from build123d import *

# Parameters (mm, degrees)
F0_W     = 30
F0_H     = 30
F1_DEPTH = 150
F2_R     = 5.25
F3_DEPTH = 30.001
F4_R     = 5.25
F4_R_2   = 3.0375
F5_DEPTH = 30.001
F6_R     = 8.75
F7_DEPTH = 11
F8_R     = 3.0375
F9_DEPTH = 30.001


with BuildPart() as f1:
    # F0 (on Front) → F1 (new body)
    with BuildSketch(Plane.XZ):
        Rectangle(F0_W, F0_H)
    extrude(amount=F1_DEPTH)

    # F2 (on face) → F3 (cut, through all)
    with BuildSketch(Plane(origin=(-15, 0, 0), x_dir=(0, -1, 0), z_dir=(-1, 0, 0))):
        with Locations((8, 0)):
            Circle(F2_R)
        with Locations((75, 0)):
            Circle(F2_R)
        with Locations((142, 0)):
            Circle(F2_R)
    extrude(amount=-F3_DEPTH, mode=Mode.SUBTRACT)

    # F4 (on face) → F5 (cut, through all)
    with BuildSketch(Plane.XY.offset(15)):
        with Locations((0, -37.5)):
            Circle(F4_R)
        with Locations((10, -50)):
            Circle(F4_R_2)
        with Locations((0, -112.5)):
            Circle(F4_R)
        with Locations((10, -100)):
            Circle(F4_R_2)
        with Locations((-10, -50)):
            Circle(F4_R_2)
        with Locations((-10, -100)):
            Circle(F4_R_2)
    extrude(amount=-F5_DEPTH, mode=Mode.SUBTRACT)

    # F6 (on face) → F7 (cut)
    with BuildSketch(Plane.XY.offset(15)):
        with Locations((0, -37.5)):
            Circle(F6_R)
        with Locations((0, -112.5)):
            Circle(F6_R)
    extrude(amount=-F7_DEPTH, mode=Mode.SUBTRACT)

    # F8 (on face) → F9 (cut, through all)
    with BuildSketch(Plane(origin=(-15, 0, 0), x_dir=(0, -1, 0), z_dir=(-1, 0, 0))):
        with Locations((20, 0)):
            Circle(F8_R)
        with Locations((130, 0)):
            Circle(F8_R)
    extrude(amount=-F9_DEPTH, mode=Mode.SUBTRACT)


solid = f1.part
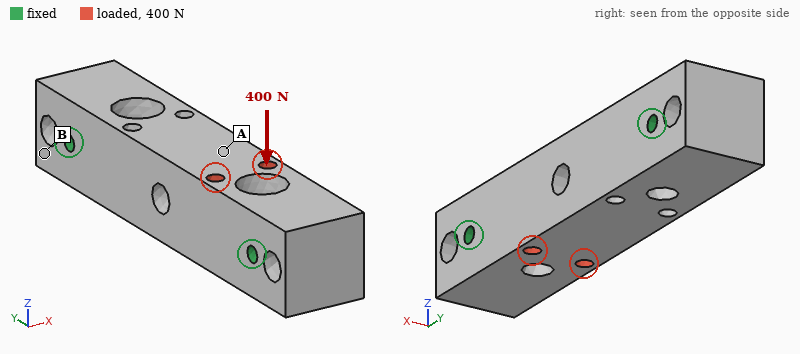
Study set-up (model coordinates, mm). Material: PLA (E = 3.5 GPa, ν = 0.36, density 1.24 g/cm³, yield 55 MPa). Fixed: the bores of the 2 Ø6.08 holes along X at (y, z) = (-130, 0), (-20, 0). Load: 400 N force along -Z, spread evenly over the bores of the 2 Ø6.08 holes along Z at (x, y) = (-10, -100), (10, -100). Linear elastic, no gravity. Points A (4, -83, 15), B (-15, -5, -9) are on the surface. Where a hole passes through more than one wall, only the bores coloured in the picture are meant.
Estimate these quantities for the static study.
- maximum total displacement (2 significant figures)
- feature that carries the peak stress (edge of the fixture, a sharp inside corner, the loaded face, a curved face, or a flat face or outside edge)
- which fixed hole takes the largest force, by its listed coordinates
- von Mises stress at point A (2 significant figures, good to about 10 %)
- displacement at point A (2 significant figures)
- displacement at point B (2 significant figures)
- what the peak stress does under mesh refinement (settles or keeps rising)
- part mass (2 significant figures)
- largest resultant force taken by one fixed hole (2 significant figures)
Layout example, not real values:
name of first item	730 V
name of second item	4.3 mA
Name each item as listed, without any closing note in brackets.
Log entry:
maximum total displacement	35 µm
feature that carries the peak stress	a sharp inside corner
which fixed hole takes the largest force, by its listed coordinates	(-130, 0)
von Mises stress at point A	0.97 MPa
displacement at point A	32 µm
displacement at point B	6.6 µm
what the peak stress does under mesh refinement	keeps rising
part mass	140 g
largest resultant force taken by one fixed hole	310 N
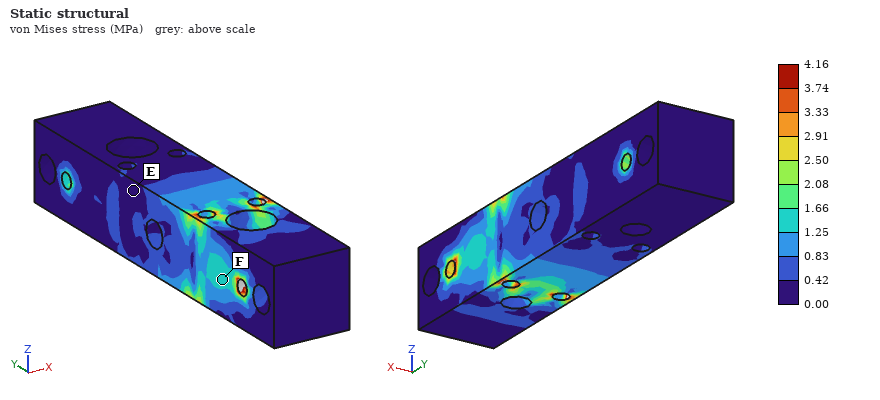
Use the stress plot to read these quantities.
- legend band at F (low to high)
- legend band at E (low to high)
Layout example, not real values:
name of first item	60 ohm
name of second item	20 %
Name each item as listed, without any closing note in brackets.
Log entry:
legend band at F	1.25 to 1.66 MPa
legend band at E	0.00 to 0.42 MPa
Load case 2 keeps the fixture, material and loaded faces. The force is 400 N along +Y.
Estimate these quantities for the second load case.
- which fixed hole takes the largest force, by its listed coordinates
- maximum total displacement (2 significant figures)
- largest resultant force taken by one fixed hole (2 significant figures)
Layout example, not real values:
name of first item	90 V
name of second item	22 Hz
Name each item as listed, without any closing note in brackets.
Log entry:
which fixed hole takes the largest force, by its listed coordinates	(-130, 0)
maximum total displacement	5.3 µm
largest resultant force taken by one fixed hole	280 N
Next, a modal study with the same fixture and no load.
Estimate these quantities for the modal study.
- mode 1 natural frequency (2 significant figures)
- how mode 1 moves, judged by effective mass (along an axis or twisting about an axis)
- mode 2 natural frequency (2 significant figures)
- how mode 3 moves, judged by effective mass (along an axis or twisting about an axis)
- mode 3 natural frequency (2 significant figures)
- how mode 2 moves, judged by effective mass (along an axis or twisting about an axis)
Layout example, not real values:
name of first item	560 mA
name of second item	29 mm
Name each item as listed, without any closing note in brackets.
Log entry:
mode 1 natural frequency	2100 Hz
how mode 1 moves, judged by effective mass	along Z
mode 2 natural frequency	2400 Hz
how mode 3 moves, judged by effective mass	twisting about Y
mode 3 natural frequency	3600 Hz
how mode 2 moves, judged by effective mass	along X
